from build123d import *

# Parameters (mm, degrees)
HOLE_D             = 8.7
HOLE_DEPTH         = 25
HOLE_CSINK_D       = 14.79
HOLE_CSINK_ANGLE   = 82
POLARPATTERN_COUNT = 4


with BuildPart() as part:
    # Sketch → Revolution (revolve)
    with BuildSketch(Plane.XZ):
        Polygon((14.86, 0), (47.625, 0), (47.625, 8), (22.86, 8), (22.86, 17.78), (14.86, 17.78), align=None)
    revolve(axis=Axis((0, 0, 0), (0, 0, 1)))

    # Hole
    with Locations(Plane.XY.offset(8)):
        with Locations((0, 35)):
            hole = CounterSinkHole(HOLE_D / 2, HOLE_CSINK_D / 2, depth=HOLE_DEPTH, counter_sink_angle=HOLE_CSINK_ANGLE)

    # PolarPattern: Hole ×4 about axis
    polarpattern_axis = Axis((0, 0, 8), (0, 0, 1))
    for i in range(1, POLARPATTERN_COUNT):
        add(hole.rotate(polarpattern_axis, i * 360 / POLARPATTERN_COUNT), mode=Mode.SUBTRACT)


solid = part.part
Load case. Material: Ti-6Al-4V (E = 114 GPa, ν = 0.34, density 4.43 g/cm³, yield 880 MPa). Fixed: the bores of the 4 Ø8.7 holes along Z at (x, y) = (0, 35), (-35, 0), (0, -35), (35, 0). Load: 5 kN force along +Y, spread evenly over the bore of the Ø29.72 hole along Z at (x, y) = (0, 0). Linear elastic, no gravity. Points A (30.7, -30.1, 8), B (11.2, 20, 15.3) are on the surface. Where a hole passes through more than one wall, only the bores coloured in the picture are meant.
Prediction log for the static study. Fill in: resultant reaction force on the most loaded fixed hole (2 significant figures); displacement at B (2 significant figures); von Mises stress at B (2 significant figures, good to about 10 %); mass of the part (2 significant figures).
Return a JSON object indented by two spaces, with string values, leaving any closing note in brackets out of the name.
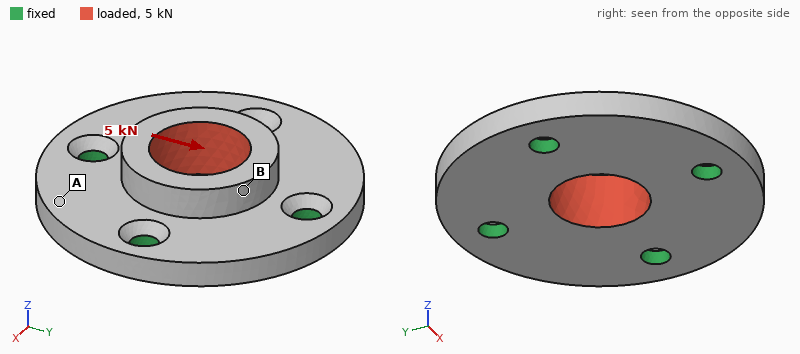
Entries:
{
  "resultant reaction force on the most loaded fixed hole": "1.6 kN",
  "displacement at B": "2.7 µm",
  "von Mises stress at B": "4.0 MPa",
  "mass of the part": "260 g"
}
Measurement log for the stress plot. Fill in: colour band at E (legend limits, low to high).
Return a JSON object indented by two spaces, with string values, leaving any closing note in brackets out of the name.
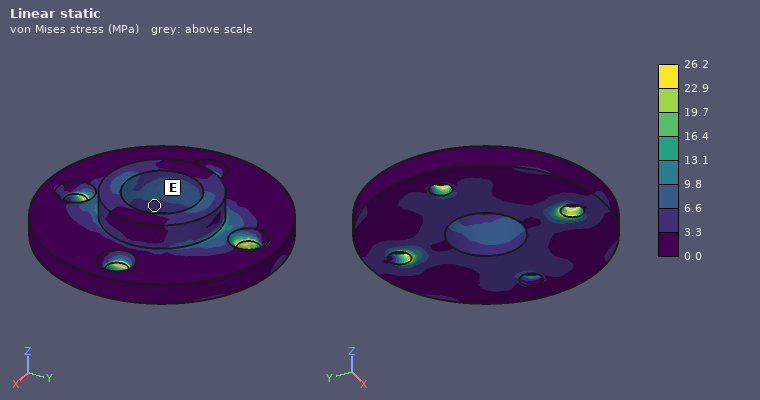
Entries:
{
  "colour band at E": "3.3 to 6.6 MPa"
}
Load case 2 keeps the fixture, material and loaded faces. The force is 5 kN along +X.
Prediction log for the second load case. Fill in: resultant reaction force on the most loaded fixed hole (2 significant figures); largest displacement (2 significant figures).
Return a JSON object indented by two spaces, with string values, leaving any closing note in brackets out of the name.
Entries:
{
  "resultant reaction force on the most loaded fixed hole": "1.6 kN",
  "largest displacement": "3.1 µm"
}
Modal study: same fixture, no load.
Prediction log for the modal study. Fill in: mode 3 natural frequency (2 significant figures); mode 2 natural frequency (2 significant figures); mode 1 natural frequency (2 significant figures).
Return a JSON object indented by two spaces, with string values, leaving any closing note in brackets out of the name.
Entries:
{
  "mode 3 natural frequency": "9900 Hz",
  "mode 2 natural frequency": "9900 Hz",
  "mode 1 natural frequency": "9100 Hz"
}
